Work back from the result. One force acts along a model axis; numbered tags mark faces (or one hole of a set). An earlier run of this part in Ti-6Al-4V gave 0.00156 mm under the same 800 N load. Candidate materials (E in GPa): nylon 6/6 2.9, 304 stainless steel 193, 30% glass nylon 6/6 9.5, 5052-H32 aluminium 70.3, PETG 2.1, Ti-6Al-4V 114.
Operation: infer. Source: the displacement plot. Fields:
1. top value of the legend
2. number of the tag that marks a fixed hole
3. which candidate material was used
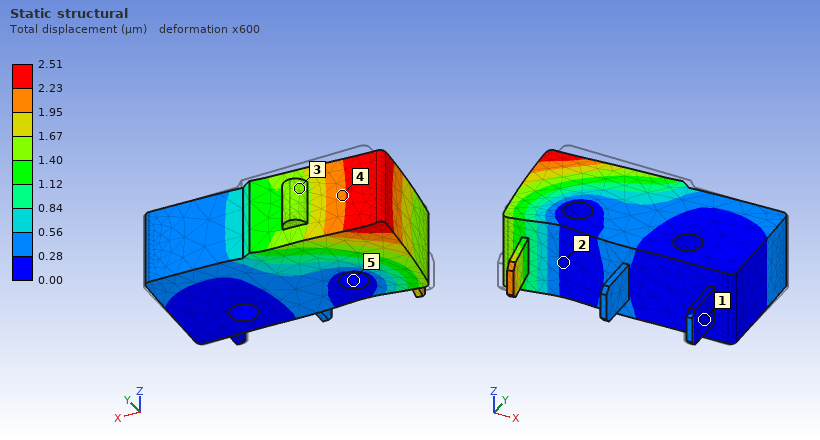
2.51 µm
5
5052-H32 aluminium
